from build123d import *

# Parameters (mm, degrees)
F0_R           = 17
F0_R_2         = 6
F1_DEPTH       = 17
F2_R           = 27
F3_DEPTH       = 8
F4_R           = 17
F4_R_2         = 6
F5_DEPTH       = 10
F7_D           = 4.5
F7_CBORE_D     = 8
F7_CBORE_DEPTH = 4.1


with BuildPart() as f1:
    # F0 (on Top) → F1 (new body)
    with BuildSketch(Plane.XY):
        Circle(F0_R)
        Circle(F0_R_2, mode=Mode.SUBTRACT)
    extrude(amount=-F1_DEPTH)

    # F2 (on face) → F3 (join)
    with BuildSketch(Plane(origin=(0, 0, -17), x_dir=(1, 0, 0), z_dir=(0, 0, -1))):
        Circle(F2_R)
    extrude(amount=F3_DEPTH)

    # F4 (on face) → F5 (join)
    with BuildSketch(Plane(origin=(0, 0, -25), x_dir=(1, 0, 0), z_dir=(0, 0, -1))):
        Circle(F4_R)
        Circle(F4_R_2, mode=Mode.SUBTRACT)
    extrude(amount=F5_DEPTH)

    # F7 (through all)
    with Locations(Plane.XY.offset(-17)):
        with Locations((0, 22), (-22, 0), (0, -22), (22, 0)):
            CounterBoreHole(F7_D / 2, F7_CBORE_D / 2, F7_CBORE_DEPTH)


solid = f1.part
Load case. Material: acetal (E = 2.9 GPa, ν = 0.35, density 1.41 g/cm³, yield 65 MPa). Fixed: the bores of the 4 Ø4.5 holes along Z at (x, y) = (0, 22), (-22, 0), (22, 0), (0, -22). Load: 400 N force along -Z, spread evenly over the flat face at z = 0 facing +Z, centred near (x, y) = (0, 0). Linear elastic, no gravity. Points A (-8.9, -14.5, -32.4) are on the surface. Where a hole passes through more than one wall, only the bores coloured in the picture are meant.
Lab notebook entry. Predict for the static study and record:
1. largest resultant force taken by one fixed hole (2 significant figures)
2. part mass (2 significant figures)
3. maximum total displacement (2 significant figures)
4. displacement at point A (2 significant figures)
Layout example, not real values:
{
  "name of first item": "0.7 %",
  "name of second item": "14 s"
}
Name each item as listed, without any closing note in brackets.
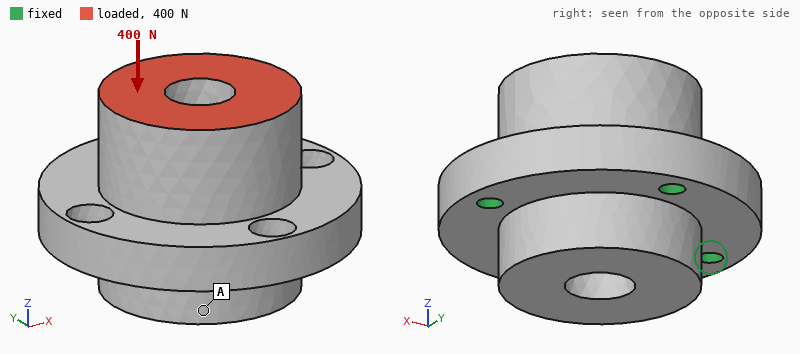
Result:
{
  "largest resultant force taken by one fixed hole": "100 N",
  "part mass": "55 g",
  "maximum total displacement": "13 µm",
  "displacement at point A": "9.9 µm"
}
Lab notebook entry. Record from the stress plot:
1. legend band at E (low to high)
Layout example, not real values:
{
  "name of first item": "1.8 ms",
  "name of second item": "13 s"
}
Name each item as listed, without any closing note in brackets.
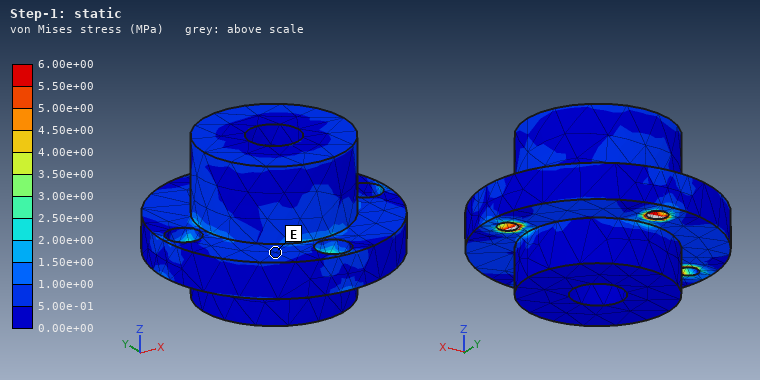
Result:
{
  "legend band at E": "5.00e-01 to 1.00e+00 MPa"
}
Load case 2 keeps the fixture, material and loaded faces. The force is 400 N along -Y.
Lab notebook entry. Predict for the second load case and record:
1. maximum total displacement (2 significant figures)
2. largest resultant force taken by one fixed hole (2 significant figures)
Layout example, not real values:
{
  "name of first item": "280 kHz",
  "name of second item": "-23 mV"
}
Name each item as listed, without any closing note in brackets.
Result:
{
  "maximum total displacement": "52 µm",
  "largest resultant force taken by one fixed hole": "260 N"
}
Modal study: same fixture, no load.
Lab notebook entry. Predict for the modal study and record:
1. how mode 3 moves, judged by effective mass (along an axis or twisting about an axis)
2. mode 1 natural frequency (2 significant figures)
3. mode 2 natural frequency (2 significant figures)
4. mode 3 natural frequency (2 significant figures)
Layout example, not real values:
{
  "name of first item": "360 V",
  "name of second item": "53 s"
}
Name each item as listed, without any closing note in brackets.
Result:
{
  "how mode 3 moves, judged by effective mass": "along Z",
  "mode 1 natural frequency": "4200 Hz",
  "mode 2 natural frequency": "4200 Hz",
  "mode 3 natural frequency": "4400 Hz"
}
